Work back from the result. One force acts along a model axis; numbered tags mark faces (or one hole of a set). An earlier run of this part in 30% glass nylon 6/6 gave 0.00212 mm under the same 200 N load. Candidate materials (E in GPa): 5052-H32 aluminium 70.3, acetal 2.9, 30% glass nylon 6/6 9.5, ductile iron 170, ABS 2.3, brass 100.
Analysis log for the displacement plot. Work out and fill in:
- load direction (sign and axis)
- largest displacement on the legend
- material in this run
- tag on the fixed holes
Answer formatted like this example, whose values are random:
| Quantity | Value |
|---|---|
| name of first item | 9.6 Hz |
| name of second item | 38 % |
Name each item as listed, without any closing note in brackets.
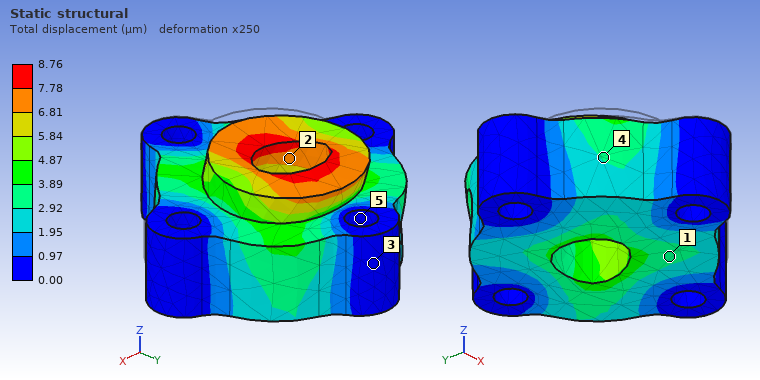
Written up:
| Quantity | Value |
|---|---|
| load direction | +Y |
| largest displacement on the legend | 8.76 µm |
| material in this run | ABS |
| tag on the fixed holes | 5 |
